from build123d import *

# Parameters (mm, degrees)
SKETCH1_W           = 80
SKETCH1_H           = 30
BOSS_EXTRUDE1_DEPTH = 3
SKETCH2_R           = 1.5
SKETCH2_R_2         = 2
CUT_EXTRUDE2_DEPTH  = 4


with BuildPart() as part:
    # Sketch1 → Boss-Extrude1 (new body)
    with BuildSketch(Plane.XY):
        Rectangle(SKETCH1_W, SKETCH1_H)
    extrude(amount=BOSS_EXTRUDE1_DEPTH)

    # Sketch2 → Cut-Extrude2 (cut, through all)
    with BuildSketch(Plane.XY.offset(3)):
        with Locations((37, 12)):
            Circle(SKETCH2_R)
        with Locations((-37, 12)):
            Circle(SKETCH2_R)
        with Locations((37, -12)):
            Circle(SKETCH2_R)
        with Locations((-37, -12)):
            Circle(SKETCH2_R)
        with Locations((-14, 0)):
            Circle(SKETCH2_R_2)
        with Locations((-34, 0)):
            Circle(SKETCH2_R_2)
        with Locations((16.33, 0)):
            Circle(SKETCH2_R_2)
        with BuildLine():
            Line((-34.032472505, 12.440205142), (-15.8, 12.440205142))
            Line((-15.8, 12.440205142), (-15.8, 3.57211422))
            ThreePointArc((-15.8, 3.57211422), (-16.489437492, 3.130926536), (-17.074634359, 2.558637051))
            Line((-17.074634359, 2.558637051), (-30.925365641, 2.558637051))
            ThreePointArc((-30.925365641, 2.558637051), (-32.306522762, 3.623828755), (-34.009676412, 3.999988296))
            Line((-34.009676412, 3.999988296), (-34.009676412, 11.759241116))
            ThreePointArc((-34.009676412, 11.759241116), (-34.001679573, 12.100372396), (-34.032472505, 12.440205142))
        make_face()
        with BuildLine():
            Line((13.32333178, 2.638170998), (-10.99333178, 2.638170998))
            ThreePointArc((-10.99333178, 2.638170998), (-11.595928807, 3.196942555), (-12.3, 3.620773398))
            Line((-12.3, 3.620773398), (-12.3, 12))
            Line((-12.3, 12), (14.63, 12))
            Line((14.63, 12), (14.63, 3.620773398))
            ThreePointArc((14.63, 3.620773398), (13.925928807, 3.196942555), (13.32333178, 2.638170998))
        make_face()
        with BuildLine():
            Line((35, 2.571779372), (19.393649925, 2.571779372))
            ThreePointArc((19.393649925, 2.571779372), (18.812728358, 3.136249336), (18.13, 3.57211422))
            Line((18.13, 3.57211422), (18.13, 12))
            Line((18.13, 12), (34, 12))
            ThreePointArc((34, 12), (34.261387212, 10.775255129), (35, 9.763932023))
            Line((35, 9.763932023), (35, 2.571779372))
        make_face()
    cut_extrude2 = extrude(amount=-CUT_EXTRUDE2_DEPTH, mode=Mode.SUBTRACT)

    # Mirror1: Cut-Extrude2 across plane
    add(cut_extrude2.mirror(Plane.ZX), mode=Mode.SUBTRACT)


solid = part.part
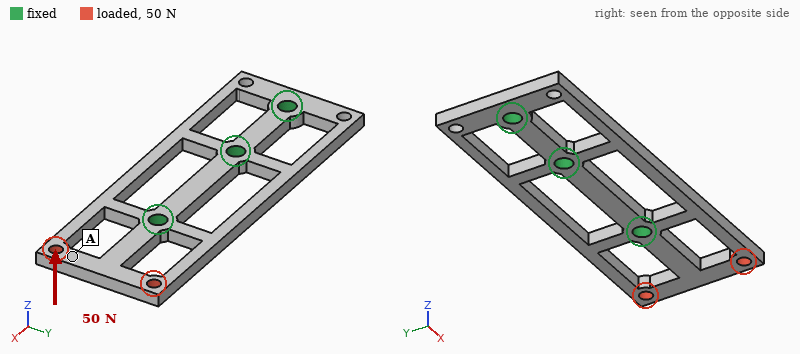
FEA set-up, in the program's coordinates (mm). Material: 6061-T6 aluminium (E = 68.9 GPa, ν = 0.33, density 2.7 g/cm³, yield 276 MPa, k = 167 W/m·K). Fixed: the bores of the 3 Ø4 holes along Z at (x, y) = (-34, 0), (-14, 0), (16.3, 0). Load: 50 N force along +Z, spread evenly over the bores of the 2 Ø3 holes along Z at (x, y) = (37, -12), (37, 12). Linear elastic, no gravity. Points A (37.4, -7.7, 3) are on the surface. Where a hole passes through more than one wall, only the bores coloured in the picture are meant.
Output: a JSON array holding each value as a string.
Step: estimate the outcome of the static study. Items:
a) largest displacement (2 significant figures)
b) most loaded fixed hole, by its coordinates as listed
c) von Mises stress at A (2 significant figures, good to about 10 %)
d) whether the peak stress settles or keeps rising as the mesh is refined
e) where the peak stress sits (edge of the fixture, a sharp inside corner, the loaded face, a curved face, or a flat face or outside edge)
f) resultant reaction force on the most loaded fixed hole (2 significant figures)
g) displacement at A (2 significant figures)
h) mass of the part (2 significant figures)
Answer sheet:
["0.12 mm", "(16.3, 0)", "9.5 MPa", "keeps rising", "edge of the fixture", "57 N", "0.098 mm", "9.5 g"]
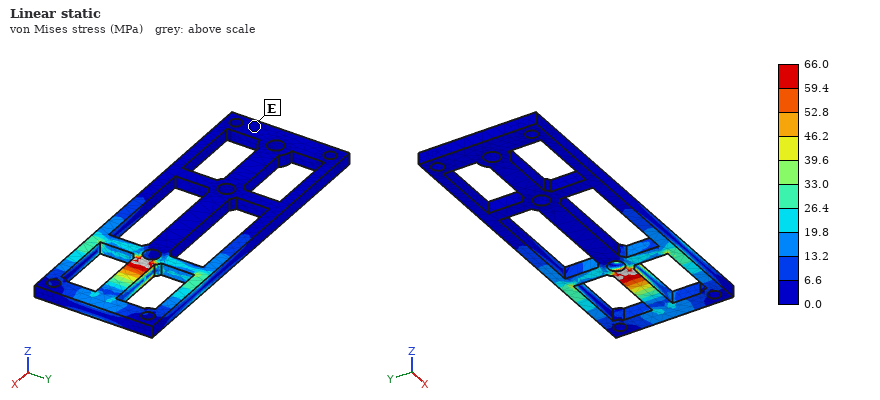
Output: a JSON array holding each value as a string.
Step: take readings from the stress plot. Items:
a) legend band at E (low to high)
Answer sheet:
["0.0 to 6.6 MPa"]
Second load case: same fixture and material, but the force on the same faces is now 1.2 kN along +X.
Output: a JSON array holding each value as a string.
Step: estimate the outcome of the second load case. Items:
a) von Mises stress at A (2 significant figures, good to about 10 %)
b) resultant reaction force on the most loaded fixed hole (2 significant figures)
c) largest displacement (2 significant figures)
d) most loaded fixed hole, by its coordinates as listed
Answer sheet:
["47 MPa", "780 N", "49 µm", "(16.3, 0)"]
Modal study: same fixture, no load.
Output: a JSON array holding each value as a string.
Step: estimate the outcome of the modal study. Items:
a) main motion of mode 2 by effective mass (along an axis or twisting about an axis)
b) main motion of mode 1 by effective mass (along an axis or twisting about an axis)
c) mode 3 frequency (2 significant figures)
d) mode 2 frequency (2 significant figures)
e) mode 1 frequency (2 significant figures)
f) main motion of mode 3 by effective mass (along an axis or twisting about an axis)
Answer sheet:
["twisting about X", "along Z", "6300 Hz", "4400 Hz", "2900 Hz", "along Z"]
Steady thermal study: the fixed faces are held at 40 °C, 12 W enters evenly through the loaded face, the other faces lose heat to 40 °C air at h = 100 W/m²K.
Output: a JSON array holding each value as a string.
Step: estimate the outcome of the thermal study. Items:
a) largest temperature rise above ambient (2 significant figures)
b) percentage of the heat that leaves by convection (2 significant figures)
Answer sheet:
["44 K", "31 %"]
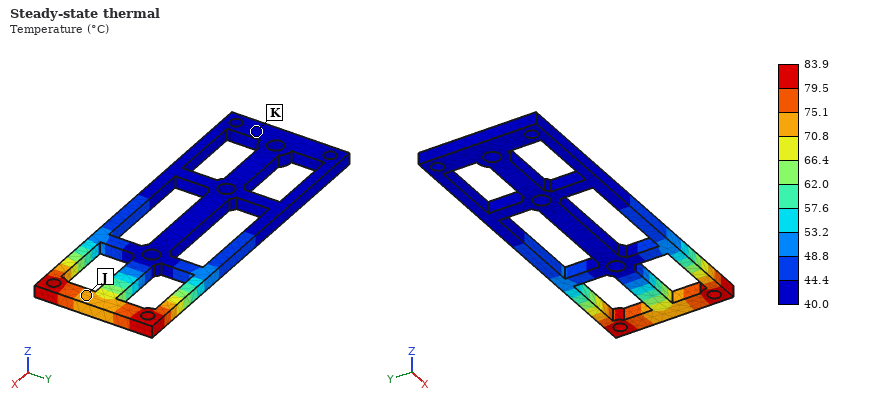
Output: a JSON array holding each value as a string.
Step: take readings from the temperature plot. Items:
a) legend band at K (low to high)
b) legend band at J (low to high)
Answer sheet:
["40.0 to 44.4 °C", "70.8 to 75.1 °C"]
